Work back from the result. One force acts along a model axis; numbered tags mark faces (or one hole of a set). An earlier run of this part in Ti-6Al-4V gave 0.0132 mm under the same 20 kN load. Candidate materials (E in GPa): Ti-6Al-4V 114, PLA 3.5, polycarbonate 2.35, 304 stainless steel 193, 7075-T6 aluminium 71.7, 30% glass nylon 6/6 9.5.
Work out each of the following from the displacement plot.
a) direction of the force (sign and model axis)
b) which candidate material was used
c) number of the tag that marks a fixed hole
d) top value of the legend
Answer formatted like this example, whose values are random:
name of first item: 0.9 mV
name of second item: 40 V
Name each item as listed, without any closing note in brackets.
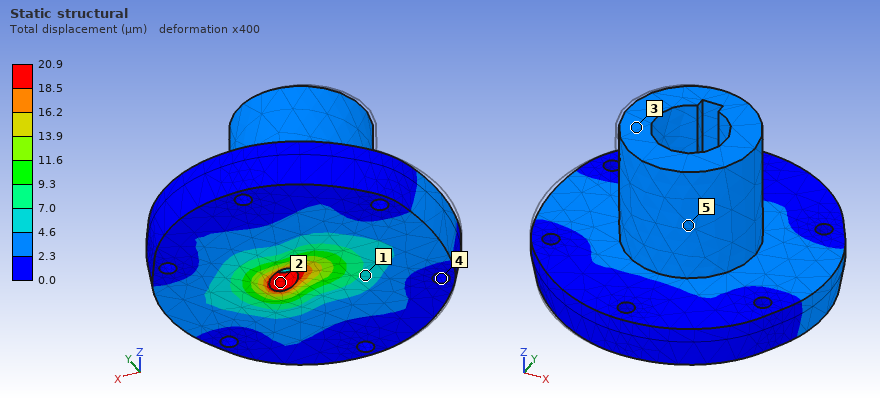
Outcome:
direction of the force: +X
which candidate material was used: 7075-T6 aluminium
number of the tag that marks a fixed hole: 4
top value of the legend: 20.9 µm
